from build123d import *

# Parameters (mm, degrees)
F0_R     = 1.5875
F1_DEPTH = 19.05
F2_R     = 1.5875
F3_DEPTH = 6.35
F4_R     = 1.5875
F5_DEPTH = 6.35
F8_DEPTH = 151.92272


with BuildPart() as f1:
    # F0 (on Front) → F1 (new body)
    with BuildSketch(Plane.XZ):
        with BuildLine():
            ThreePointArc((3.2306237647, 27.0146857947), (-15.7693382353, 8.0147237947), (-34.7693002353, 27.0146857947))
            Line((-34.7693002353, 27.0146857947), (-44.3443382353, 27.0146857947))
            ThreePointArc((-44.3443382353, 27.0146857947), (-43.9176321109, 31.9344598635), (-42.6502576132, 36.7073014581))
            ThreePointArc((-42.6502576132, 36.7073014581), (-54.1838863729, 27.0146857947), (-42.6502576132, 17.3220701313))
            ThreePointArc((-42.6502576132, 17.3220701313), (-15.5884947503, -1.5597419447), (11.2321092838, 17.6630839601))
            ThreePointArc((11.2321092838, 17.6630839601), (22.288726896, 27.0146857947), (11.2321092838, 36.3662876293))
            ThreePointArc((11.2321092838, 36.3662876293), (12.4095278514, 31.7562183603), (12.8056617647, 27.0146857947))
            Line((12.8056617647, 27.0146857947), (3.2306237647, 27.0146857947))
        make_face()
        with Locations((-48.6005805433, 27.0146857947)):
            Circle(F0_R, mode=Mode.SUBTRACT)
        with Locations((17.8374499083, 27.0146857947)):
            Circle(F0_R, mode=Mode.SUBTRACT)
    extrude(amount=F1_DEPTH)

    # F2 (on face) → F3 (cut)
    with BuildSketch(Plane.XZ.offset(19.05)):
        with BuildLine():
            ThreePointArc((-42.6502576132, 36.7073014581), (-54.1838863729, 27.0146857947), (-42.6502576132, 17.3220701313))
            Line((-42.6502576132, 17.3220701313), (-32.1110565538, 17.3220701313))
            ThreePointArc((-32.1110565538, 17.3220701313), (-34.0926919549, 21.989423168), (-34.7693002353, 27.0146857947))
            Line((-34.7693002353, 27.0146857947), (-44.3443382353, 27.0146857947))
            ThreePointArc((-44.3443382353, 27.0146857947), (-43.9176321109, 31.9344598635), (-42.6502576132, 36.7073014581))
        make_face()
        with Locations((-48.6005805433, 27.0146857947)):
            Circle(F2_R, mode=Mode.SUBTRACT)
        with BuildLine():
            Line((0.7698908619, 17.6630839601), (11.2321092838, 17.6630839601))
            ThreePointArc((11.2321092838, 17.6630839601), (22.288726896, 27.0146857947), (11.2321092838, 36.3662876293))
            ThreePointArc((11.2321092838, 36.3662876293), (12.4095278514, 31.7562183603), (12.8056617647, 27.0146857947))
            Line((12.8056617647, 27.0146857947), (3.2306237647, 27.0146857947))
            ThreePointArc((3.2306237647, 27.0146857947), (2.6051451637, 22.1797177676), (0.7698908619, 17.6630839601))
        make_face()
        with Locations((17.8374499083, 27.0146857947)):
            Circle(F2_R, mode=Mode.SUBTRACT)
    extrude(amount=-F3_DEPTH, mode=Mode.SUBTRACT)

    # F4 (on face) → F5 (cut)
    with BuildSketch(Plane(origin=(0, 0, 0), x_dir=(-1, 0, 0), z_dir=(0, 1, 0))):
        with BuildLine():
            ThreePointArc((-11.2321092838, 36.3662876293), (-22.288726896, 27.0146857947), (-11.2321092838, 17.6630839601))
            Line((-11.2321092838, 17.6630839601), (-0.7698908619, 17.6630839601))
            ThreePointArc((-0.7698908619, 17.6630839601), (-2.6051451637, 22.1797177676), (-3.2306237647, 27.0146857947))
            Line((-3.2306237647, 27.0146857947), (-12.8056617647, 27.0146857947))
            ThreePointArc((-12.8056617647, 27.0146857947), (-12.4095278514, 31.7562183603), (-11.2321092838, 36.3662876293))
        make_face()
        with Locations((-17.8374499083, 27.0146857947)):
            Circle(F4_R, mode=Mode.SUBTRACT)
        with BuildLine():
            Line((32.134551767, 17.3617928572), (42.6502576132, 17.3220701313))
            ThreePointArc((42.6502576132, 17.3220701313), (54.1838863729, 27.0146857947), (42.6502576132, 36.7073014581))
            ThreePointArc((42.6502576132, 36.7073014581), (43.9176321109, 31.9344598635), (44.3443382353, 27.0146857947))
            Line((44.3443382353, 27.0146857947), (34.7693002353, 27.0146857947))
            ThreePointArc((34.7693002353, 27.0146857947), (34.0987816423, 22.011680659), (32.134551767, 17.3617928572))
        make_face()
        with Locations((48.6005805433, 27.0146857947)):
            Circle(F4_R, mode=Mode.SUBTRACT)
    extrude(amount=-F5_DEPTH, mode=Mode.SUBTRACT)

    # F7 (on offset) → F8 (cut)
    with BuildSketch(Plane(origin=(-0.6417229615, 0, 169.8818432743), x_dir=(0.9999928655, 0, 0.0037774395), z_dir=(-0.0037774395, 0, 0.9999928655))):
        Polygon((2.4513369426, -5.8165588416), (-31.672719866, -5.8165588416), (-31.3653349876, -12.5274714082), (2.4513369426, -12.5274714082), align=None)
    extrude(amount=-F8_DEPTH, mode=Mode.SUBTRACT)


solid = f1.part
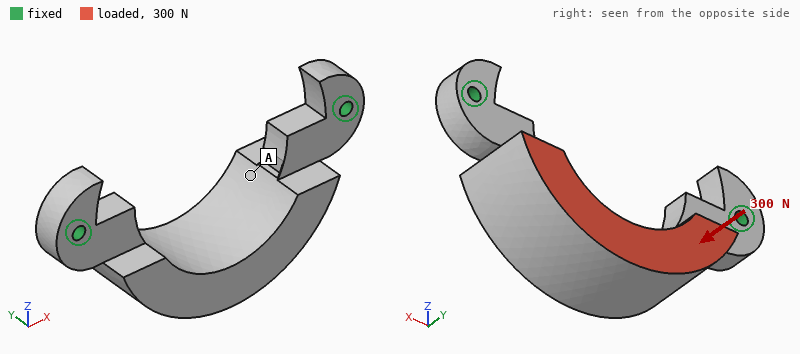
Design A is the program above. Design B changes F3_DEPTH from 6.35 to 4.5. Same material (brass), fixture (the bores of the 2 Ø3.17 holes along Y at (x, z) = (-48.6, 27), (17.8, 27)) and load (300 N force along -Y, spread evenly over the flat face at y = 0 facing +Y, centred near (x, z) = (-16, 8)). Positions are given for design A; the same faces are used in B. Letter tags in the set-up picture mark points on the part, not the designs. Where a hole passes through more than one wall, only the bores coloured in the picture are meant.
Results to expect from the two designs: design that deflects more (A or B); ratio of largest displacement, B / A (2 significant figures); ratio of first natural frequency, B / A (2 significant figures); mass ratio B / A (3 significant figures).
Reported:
A
0.56
1.3
1.07
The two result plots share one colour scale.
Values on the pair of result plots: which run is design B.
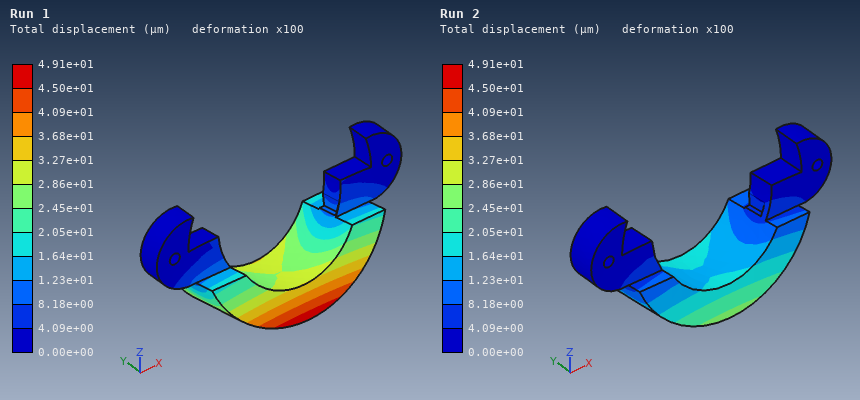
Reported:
Run 2
